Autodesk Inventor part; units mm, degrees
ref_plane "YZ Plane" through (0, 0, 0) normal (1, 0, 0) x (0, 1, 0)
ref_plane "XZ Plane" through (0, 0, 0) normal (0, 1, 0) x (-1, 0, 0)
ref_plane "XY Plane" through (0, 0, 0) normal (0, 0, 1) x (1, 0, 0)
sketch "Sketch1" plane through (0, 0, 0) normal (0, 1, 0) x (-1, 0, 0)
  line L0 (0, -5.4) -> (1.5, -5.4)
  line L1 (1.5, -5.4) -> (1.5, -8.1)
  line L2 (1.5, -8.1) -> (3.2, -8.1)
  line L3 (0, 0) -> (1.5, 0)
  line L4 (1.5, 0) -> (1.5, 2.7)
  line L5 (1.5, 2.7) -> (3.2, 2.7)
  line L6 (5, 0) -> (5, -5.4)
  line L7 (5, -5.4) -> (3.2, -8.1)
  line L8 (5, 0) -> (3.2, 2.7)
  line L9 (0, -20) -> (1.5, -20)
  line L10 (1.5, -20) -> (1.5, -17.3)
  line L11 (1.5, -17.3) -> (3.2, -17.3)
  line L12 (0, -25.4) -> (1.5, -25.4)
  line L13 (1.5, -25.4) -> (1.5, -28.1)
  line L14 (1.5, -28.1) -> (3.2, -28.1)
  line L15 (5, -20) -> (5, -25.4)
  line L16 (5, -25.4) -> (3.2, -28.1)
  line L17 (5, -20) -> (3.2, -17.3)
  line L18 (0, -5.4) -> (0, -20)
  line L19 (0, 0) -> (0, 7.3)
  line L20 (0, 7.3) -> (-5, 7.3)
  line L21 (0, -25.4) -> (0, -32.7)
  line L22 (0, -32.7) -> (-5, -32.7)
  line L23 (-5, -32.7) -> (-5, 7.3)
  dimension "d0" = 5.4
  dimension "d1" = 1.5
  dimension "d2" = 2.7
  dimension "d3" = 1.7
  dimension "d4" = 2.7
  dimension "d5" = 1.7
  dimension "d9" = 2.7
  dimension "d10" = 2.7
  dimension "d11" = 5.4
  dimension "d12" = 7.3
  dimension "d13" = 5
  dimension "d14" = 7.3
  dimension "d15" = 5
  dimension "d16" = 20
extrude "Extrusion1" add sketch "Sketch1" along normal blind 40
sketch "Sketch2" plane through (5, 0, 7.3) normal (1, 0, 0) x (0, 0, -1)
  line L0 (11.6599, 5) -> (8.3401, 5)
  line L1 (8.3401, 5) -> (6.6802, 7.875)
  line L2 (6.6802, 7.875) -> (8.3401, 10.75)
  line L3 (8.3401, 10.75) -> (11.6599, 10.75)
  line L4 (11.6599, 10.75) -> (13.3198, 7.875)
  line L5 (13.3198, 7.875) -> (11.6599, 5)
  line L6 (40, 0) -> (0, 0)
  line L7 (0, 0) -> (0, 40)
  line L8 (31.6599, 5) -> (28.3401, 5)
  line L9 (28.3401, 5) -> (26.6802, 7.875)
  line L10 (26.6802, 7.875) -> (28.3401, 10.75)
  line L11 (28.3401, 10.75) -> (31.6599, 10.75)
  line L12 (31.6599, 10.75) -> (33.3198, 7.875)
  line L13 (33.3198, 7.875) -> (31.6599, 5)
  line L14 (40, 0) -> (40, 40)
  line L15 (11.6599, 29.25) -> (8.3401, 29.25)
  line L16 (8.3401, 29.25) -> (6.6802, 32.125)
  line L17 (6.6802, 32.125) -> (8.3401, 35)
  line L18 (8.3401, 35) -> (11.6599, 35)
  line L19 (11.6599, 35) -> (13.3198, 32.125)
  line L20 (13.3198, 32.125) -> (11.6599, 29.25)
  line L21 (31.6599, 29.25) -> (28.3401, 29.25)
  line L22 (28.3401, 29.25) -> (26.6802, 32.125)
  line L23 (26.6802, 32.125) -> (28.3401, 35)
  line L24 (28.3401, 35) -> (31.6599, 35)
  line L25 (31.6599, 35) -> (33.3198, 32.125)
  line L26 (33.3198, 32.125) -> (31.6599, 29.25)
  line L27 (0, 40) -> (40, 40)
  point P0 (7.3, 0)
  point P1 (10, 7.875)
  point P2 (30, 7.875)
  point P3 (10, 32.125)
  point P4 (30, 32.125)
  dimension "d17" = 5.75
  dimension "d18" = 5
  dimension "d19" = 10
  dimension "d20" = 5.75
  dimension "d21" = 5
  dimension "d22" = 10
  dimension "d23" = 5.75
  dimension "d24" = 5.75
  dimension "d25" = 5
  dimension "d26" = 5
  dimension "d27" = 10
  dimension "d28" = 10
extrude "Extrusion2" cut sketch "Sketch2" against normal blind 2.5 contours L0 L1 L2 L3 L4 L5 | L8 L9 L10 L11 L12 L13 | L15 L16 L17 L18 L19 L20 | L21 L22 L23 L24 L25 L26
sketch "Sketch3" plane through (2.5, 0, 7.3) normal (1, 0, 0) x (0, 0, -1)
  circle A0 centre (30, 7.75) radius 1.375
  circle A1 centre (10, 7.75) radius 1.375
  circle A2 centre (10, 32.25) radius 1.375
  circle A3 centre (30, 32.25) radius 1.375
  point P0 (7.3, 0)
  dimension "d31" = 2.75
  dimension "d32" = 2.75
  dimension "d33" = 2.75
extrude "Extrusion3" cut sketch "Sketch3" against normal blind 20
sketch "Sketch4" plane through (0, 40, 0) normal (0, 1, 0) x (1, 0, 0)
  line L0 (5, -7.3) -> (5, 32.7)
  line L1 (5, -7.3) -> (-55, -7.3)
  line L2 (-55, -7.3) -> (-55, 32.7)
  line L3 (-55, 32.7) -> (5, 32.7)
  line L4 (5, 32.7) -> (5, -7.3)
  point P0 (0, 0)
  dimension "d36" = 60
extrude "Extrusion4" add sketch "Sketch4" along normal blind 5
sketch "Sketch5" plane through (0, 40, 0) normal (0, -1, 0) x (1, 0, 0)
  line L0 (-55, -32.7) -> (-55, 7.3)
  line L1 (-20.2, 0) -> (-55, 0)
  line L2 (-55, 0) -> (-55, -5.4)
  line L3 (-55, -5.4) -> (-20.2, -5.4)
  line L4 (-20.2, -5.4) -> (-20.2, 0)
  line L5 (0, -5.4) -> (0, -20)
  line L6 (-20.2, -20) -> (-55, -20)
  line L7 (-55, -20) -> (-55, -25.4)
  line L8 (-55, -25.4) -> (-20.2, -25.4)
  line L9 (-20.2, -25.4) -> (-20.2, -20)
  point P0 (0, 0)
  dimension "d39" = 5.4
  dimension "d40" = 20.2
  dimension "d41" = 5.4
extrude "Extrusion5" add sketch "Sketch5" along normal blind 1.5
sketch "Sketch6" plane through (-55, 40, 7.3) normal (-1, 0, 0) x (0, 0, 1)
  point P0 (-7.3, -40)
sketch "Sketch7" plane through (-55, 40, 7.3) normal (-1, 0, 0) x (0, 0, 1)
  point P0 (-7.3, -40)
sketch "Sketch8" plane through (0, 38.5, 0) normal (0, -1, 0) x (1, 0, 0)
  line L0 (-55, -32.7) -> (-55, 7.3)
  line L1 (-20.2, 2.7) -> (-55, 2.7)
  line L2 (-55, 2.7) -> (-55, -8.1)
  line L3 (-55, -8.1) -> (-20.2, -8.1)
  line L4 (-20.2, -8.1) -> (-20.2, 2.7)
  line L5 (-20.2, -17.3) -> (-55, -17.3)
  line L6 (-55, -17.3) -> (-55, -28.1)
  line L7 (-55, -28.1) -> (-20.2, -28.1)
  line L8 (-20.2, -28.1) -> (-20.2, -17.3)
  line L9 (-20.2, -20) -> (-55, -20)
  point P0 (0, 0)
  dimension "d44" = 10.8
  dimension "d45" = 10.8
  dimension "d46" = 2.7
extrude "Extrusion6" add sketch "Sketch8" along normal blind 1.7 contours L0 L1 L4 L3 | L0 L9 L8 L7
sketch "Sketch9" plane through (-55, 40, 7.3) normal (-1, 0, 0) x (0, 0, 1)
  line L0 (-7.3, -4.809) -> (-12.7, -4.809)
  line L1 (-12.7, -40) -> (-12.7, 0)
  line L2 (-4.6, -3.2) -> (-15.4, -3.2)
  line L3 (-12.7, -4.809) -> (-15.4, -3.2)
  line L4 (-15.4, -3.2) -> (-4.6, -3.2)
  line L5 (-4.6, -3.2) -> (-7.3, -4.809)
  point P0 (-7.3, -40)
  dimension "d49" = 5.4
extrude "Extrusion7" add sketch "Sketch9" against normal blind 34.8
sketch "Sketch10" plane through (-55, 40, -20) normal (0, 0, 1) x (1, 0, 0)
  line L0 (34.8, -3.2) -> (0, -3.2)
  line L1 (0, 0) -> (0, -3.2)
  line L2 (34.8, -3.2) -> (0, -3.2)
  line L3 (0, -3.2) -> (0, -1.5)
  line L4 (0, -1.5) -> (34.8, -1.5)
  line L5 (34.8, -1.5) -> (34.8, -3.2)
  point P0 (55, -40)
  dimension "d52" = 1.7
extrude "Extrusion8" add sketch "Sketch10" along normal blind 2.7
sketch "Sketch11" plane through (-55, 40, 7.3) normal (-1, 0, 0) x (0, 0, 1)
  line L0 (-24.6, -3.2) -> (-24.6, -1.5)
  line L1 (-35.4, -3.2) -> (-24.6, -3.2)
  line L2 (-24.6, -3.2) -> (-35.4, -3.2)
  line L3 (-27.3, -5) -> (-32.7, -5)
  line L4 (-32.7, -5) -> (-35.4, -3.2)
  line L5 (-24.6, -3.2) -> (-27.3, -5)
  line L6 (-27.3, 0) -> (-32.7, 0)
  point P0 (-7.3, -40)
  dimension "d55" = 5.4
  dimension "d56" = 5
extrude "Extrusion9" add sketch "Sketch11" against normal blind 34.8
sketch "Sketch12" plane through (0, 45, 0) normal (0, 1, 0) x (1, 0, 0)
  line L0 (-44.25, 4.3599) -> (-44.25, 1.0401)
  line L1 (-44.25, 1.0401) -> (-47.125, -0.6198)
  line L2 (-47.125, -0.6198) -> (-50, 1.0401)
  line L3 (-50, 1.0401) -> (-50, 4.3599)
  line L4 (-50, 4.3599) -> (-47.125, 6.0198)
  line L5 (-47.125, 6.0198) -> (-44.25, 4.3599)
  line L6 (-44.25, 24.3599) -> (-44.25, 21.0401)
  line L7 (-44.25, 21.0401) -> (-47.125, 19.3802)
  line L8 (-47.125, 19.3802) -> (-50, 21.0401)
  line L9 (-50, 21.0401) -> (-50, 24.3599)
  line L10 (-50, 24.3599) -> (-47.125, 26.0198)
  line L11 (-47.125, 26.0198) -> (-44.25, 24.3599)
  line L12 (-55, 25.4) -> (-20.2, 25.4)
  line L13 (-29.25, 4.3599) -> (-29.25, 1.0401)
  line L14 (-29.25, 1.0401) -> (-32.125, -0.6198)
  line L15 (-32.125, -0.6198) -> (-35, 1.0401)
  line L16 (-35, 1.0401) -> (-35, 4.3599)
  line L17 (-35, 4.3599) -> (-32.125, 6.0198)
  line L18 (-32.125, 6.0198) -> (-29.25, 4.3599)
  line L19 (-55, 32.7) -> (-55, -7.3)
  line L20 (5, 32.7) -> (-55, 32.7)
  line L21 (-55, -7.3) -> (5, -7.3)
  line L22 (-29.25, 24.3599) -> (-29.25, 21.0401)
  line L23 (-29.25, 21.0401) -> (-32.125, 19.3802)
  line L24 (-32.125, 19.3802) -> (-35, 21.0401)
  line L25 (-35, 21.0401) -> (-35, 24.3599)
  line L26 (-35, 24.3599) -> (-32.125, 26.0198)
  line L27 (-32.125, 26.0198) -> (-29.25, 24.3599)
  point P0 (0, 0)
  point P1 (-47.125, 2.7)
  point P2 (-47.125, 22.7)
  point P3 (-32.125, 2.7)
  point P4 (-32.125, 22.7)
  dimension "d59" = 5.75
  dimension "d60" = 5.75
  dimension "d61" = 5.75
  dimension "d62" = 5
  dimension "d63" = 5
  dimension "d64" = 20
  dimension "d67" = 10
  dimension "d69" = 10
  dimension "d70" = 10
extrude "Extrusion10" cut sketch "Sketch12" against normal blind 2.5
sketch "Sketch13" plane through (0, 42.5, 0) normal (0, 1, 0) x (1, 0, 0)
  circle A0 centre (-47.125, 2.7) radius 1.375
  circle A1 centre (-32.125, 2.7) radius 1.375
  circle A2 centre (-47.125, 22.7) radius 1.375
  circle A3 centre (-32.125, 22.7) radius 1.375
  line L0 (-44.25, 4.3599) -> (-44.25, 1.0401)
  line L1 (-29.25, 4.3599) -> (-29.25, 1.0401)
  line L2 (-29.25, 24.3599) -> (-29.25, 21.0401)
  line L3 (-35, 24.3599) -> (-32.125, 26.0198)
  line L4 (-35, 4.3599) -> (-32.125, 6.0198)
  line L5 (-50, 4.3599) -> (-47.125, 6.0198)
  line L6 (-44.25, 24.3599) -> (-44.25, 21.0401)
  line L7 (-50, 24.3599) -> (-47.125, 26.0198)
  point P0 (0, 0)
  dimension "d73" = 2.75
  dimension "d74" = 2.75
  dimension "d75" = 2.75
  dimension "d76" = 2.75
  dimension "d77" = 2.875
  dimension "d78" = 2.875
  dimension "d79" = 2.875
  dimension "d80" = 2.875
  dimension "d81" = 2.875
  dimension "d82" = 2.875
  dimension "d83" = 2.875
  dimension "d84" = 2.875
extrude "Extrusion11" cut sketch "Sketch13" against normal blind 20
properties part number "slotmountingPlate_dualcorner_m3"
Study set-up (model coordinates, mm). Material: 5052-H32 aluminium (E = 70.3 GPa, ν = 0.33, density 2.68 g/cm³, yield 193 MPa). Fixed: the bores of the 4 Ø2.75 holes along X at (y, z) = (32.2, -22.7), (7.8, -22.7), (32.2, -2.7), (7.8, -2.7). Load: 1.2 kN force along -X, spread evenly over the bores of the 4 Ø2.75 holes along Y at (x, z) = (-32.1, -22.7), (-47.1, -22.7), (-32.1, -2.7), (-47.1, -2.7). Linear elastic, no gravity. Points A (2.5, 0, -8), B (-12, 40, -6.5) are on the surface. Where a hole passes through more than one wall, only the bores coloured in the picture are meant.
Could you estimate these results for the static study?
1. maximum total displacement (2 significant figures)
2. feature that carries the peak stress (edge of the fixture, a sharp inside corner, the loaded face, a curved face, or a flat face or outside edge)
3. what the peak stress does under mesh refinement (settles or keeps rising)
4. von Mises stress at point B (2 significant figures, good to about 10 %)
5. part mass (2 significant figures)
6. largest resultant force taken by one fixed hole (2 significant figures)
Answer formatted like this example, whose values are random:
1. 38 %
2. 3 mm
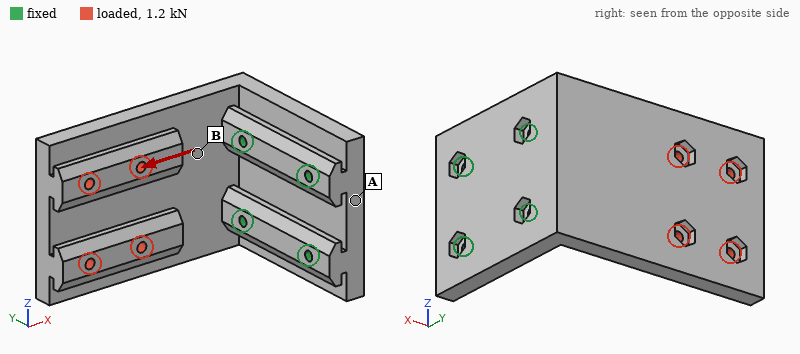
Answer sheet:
1. 0.12 mm
2. edge of the fixture
3. keeps rising
4. 30 MPa
5. 67 g
6. 670 N
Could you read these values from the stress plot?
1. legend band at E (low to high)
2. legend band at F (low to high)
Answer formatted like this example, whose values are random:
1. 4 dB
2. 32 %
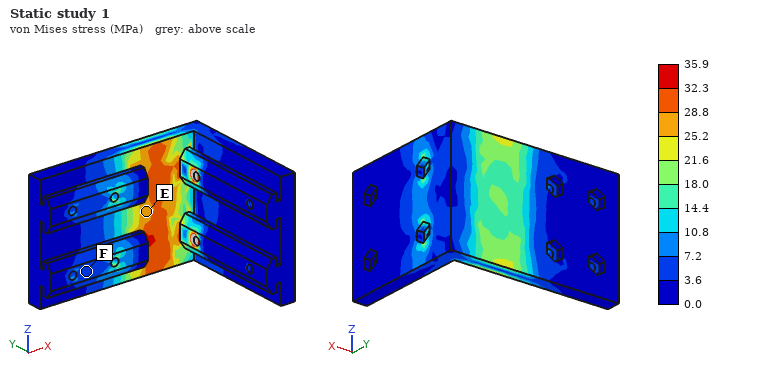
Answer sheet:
1. 25.2 to 28.8 MPa
2. 3.6 to 7.2 MPa
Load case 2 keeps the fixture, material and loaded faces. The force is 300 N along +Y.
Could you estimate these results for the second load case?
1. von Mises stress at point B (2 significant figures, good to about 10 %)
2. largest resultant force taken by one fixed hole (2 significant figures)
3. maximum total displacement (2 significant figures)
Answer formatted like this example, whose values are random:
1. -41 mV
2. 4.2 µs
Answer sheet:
1. 44 MPa
2. 380 N
3. 0.32 mm
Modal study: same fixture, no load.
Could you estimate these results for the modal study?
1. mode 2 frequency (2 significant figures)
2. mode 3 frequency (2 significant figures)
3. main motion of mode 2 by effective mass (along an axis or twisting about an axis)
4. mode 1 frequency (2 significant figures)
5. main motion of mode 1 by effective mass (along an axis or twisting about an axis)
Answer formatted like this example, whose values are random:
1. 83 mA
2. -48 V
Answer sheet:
1. 3200 Hz
2. 4100 Hz
3. along Z
4. 1200 Hz
5. along Y
